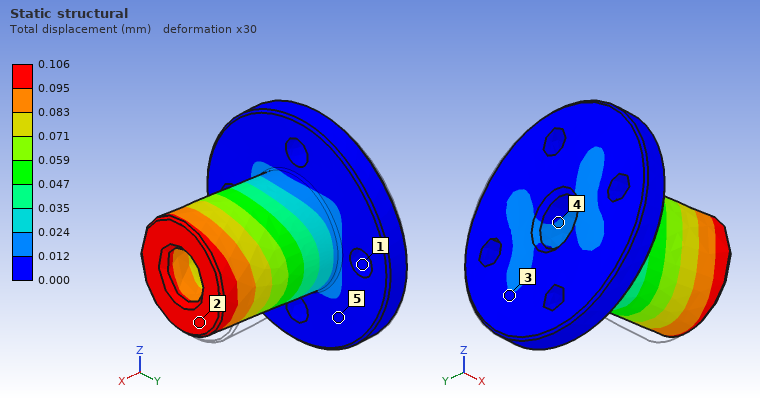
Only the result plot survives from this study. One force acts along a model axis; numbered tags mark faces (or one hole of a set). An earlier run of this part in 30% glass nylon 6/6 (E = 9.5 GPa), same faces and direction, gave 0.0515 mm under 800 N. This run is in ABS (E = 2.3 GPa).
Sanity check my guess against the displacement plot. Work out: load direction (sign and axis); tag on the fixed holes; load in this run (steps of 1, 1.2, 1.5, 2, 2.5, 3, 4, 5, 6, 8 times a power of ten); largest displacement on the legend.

-Y
1
400 N
0.106 mm
